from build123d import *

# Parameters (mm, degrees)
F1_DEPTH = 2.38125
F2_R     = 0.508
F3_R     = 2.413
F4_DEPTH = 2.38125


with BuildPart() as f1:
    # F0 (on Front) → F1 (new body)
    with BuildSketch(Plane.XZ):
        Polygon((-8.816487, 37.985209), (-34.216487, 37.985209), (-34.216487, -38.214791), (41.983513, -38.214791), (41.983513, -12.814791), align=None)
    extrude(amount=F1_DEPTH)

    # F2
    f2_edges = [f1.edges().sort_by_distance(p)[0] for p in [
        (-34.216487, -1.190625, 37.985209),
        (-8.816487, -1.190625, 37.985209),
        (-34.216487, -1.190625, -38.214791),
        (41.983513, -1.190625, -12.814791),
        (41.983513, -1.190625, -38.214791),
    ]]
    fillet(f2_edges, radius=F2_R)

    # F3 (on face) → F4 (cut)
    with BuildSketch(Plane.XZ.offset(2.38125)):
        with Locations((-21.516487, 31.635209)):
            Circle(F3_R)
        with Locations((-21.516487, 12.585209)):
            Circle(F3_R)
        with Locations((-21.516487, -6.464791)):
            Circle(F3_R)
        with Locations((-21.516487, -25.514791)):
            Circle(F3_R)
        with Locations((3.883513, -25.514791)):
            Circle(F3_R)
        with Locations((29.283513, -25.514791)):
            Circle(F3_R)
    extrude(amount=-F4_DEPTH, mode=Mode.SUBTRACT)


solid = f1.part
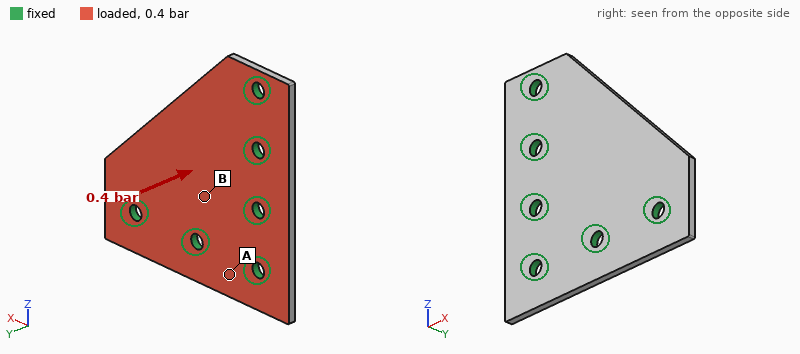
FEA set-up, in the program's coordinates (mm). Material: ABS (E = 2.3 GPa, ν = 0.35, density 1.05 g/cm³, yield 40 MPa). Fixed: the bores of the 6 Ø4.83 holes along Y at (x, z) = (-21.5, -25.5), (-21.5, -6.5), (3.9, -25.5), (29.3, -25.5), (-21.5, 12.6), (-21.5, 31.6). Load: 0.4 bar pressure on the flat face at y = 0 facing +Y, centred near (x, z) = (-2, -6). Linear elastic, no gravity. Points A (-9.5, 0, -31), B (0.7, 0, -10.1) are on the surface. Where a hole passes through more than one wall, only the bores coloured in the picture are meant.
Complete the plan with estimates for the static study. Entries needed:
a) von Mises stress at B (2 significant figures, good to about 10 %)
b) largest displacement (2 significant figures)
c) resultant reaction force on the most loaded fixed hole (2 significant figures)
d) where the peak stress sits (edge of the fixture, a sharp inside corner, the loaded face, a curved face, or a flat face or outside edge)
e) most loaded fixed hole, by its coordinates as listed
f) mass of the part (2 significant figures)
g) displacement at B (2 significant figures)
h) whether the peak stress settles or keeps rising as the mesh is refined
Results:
4.1 MPa
1.1 mm
41 N
edge of the fixture
(29.3, -25.5)
11 g
0.20 mm
keeps rising
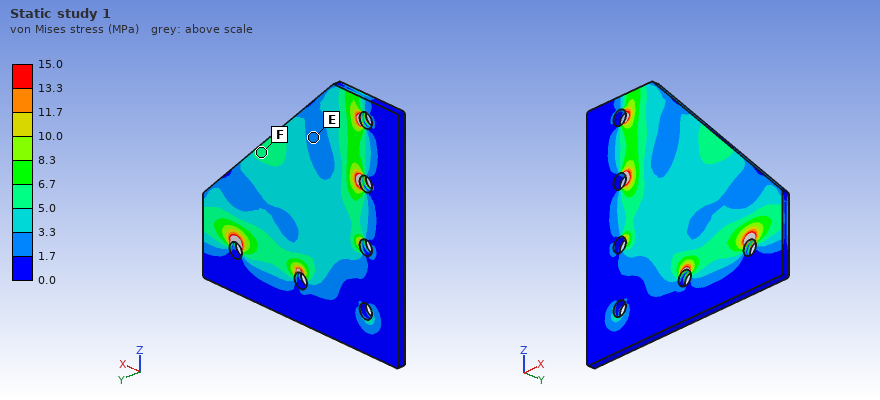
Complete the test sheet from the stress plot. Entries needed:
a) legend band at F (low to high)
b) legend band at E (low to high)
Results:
5.0 to 6.7 MPa
1.7 to 3.3 MPa
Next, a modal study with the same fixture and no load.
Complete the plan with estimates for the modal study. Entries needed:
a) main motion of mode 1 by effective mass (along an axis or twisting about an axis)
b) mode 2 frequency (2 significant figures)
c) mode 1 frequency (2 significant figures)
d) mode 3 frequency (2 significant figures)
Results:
along Y
1800 Hz
840 Hz
2500 Hz
